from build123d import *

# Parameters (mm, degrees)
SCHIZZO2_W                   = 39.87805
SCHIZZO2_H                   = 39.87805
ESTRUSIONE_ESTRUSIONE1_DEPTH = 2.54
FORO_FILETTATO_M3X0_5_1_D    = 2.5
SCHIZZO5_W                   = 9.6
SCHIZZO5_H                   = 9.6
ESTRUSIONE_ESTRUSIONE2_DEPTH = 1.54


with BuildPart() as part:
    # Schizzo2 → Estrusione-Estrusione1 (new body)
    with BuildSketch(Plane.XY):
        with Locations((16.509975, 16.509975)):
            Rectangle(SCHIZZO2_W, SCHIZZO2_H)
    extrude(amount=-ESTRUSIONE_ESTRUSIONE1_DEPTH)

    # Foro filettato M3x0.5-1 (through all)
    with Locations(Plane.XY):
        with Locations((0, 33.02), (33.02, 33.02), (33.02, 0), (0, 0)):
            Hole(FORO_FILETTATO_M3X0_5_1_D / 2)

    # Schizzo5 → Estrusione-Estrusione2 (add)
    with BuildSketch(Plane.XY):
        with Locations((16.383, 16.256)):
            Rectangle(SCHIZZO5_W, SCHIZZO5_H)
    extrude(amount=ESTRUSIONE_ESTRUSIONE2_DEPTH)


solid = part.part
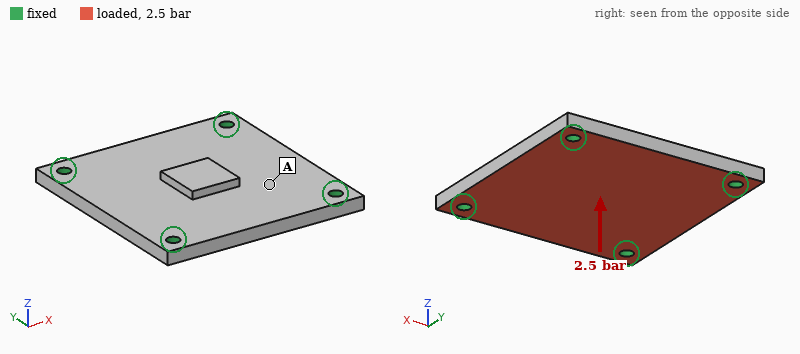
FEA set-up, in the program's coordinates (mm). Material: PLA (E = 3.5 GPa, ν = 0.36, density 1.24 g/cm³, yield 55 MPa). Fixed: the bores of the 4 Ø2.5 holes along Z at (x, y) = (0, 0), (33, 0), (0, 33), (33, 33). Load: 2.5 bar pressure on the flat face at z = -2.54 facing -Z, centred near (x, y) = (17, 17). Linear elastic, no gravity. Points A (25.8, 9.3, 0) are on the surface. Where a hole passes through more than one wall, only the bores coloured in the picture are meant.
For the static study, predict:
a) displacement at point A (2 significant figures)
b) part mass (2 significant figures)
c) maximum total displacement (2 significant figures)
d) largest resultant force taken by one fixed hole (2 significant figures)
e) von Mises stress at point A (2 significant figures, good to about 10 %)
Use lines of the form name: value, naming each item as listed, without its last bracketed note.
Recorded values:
displacement at point A: 0.26 mm
part mass: 5.1 g
maximum total displacement: 0.35 mm
largest resultant force taken by one fixed hole: 98 N
von Mises stress at point A: 9.0 MPa
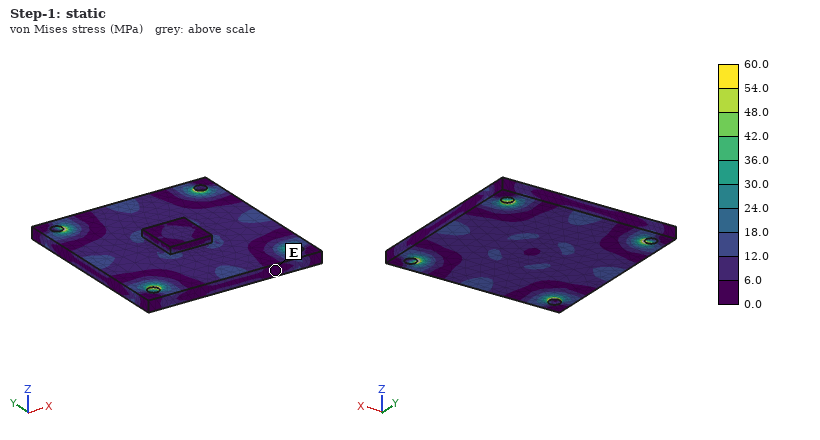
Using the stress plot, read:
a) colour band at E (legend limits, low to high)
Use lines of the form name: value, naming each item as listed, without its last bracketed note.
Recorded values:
colour band at E: 0.0 to 6.0 MPa
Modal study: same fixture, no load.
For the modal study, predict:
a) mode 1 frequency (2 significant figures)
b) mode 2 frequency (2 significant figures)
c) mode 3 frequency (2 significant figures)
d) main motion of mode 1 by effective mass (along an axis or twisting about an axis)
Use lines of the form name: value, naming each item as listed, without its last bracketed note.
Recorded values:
mode 1 frequency: 2700 Hz
mode 2 frequency: 4400 Hz
mode 3 frequency: 4400 Hz
main motion of mode 1 by effective mass: along Z
